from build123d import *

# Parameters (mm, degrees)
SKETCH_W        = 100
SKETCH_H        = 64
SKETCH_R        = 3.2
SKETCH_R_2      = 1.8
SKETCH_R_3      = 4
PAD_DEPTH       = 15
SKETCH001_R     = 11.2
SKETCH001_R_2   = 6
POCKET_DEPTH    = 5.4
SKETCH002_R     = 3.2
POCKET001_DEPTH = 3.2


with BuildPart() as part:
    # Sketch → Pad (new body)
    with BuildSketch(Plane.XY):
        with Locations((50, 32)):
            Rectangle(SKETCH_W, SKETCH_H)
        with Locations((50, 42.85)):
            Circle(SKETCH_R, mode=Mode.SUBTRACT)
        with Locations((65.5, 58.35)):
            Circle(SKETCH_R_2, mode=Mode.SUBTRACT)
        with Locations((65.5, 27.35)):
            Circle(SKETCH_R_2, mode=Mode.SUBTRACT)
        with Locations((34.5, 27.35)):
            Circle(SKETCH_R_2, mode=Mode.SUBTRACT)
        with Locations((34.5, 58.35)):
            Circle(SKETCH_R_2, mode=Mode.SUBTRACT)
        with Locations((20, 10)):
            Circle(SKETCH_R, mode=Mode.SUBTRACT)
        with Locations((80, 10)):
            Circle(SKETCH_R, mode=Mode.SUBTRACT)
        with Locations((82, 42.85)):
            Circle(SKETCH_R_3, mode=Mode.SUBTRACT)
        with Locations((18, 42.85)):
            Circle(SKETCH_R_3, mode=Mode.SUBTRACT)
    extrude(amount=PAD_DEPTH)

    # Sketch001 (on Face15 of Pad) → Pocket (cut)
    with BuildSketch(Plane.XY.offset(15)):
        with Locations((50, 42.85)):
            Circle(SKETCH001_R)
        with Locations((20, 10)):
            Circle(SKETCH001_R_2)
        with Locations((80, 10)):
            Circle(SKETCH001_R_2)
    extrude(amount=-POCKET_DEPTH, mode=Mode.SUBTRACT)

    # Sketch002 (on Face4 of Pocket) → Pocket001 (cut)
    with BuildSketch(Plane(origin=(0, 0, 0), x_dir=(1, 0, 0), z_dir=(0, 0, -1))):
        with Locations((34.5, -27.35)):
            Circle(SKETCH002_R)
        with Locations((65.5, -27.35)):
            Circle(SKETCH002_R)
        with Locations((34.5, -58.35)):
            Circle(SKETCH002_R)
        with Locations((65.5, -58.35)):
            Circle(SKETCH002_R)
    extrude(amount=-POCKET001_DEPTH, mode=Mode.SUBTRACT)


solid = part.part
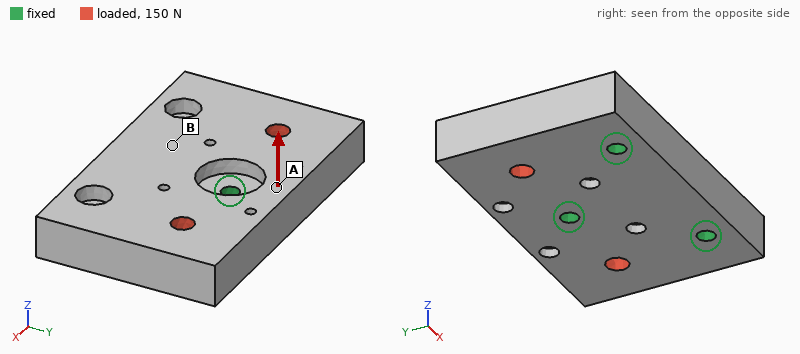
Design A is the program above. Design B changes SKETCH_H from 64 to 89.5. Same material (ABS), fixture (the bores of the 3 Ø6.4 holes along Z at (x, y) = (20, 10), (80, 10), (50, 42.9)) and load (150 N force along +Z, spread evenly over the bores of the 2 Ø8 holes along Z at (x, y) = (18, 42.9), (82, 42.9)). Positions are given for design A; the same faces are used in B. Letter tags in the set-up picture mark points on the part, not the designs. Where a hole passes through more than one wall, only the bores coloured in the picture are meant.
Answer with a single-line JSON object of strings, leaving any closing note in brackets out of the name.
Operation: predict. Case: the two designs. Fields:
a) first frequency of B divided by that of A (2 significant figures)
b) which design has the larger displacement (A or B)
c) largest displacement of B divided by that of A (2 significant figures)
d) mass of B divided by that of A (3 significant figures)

{"first frequency of B divided by that of A": "0.80", "which design has the larger displacement": "A", "largest displacement of B divided by that of A": "0.87", "mass of B divided by that of A": "1.43"}
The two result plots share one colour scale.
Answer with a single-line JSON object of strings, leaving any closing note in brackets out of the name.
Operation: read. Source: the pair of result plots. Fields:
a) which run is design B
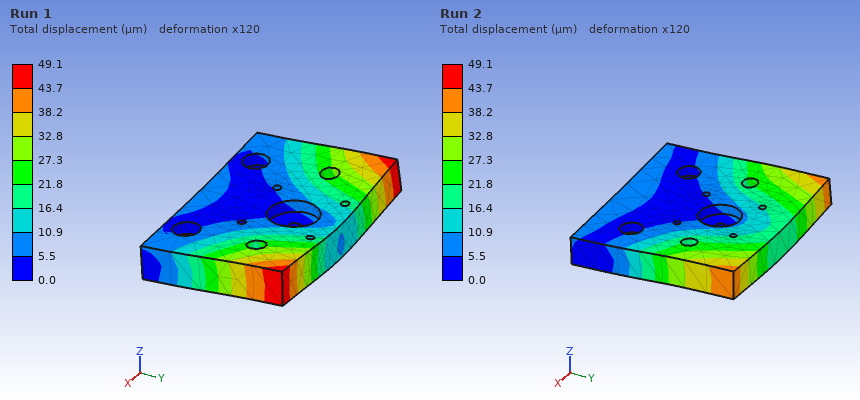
{"which run is design B": "Run 2"}
